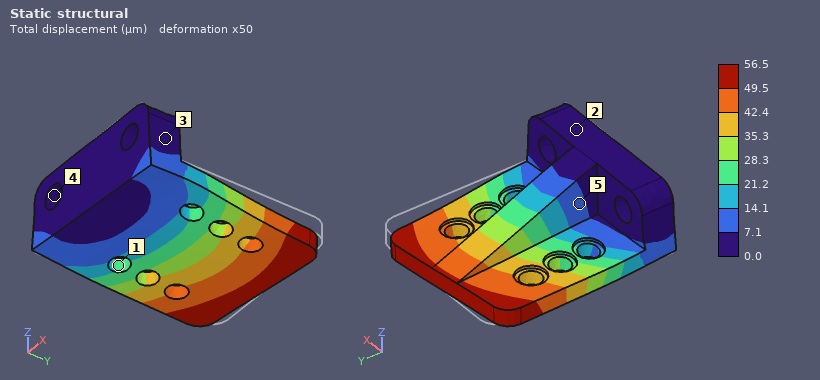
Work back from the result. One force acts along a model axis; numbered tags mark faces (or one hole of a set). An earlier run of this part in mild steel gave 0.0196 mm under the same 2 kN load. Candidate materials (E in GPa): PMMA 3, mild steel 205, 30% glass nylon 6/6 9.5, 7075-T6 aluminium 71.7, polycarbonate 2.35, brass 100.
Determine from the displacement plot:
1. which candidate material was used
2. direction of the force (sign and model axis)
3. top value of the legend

7075-T6 aluminium
-X
56.5 µm
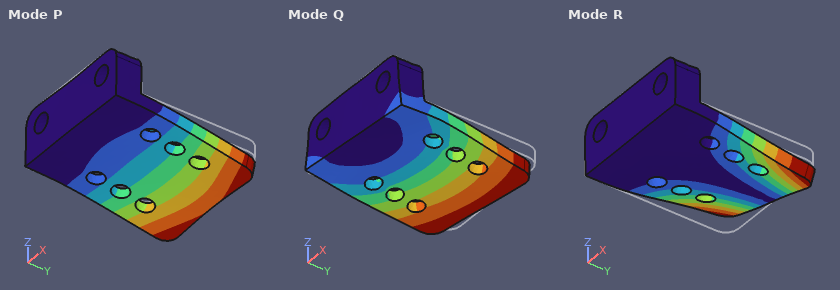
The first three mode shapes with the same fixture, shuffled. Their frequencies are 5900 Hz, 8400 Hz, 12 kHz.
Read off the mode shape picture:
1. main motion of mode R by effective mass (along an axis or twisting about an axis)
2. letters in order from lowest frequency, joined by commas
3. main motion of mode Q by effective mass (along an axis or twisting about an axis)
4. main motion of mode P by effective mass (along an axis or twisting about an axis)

twisting about Y
P, R, Q
along X
along Z
